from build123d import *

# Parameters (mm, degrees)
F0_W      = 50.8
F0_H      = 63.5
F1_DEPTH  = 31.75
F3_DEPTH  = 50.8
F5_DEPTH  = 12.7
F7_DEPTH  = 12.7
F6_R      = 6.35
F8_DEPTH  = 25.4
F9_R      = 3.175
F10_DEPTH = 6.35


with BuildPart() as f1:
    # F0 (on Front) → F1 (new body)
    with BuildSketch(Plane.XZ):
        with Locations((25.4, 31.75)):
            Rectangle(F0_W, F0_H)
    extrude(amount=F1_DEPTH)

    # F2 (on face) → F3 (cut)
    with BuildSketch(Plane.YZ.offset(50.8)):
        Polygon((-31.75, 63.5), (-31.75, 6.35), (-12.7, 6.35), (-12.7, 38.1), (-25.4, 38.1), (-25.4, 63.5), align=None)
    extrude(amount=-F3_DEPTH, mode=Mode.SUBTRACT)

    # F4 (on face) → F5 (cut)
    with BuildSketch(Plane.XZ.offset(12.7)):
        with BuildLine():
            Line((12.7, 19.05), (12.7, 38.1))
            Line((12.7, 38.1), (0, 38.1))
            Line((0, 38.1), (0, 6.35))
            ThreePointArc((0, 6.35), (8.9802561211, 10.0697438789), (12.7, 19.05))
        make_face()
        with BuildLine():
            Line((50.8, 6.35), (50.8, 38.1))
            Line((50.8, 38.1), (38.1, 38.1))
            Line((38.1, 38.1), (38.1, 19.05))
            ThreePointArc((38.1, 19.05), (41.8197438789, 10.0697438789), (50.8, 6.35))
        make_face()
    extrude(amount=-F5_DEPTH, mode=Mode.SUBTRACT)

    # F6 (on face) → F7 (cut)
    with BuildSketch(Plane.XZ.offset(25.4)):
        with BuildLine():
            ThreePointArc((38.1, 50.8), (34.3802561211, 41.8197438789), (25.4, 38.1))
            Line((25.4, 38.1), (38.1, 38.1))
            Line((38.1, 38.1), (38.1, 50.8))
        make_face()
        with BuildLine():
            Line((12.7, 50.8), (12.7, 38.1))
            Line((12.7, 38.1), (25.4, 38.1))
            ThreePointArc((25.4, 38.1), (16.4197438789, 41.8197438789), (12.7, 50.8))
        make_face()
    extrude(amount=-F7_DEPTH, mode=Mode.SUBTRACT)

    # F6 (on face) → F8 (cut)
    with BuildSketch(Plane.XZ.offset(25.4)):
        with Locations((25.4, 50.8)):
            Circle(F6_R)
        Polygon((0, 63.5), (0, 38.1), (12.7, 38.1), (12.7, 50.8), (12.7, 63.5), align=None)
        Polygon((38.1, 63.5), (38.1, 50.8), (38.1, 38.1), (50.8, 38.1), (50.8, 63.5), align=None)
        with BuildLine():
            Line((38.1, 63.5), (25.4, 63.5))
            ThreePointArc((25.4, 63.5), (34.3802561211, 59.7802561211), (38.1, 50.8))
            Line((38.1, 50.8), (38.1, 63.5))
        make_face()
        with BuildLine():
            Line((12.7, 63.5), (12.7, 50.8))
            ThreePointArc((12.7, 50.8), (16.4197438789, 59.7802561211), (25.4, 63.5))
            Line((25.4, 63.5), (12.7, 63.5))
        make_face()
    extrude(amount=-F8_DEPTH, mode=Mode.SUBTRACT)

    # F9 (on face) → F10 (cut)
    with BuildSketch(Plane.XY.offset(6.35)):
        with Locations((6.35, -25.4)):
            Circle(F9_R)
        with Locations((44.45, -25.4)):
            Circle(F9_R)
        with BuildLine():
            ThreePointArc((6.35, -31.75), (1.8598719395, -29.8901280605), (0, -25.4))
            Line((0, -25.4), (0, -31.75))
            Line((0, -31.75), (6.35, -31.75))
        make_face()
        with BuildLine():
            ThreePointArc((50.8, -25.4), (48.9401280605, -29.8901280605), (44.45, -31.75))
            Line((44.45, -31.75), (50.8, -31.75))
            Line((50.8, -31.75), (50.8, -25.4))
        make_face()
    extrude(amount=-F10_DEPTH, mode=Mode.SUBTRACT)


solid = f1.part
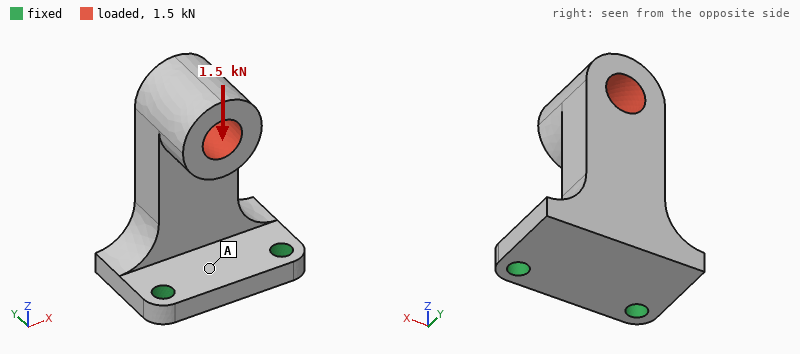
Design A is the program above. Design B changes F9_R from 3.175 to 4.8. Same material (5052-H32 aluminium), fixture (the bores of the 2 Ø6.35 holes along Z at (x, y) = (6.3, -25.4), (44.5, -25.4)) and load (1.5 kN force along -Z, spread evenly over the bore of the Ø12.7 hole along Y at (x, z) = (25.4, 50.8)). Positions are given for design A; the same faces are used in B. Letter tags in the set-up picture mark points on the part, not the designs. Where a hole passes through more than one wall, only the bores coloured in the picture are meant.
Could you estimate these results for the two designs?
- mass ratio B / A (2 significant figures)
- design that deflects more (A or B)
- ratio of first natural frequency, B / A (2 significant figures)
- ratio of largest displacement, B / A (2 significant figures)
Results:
0.98
A
1.1
0.55
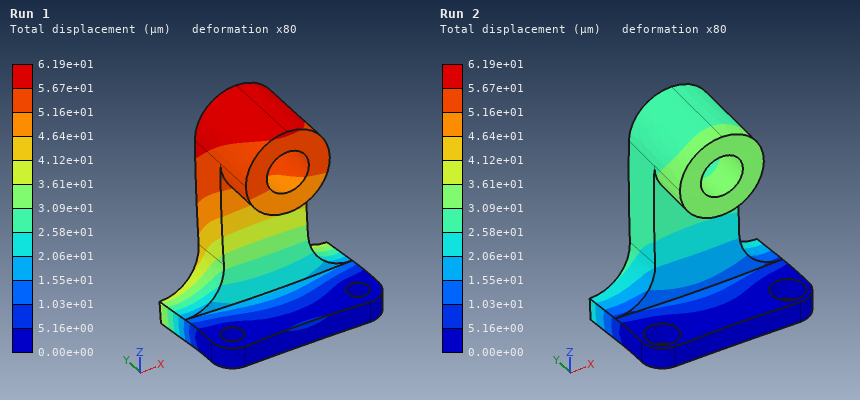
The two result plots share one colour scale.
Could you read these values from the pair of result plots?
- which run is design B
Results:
Run 2
